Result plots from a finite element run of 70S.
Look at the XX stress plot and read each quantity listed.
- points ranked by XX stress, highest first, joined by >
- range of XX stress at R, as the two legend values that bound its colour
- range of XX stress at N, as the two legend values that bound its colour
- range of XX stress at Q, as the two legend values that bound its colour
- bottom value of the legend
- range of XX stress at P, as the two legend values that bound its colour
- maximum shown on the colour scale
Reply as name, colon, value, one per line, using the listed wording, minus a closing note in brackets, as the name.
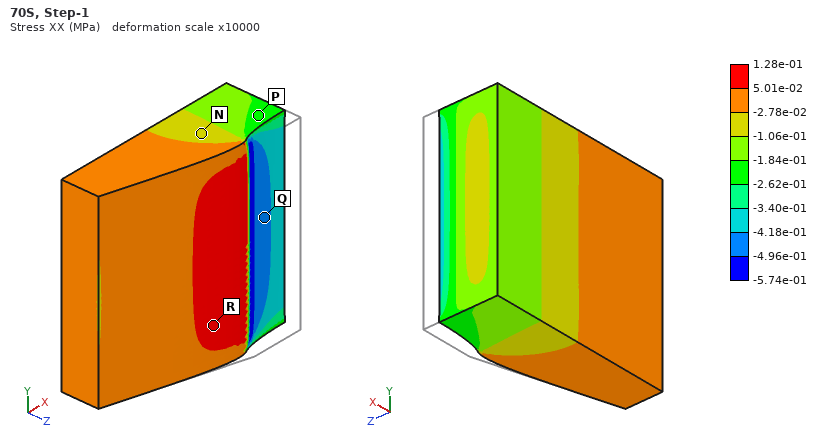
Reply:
points ranked by XX stress, highest first, joined by >: R > N > P > Q
range of XX stress at R, as the two legend values that bound its colour: 5.01e-02 to 1.28e-01 MPa
range of XX stress at N, as the two legend values that bound its colour: -1.06e-01 to -2.78e-02 MPa
range of XX stress at Q, as the two legend values that bound its colour: -4.96e-01 to -4.18e-01 MPa
bottom value of the legend: -5.74e-01 MPa
range of XX stress at P, as the two legend values that bound its colour: -2.62e-01 to -1.84e-01 MPa
maximum shown on the colour scale: 1.28e-01 MPa
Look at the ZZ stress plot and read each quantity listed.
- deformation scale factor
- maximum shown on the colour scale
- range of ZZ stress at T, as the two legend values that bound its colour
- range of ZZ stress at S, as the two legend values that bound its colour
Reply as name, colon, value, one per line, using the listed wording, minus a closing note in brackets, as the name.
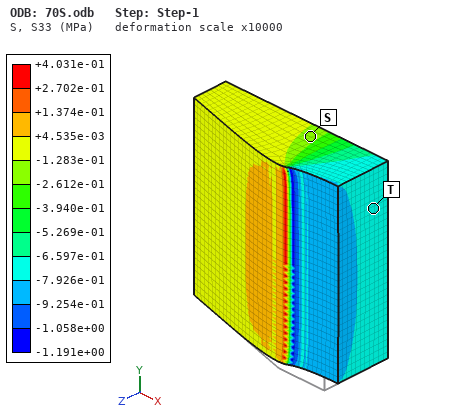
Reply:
deformation scale factor: 10000
maximum shown on the colour scale: +4.031e-01 MPa
range of ZZ stress at T, as the two legend values that bound its colour: -7.926e-01 to -6.597e-01 MPa
range of ZZ stress at S, as the two legend values that bound its colour: -2.612e-01 to -1.283e-01 MPa
